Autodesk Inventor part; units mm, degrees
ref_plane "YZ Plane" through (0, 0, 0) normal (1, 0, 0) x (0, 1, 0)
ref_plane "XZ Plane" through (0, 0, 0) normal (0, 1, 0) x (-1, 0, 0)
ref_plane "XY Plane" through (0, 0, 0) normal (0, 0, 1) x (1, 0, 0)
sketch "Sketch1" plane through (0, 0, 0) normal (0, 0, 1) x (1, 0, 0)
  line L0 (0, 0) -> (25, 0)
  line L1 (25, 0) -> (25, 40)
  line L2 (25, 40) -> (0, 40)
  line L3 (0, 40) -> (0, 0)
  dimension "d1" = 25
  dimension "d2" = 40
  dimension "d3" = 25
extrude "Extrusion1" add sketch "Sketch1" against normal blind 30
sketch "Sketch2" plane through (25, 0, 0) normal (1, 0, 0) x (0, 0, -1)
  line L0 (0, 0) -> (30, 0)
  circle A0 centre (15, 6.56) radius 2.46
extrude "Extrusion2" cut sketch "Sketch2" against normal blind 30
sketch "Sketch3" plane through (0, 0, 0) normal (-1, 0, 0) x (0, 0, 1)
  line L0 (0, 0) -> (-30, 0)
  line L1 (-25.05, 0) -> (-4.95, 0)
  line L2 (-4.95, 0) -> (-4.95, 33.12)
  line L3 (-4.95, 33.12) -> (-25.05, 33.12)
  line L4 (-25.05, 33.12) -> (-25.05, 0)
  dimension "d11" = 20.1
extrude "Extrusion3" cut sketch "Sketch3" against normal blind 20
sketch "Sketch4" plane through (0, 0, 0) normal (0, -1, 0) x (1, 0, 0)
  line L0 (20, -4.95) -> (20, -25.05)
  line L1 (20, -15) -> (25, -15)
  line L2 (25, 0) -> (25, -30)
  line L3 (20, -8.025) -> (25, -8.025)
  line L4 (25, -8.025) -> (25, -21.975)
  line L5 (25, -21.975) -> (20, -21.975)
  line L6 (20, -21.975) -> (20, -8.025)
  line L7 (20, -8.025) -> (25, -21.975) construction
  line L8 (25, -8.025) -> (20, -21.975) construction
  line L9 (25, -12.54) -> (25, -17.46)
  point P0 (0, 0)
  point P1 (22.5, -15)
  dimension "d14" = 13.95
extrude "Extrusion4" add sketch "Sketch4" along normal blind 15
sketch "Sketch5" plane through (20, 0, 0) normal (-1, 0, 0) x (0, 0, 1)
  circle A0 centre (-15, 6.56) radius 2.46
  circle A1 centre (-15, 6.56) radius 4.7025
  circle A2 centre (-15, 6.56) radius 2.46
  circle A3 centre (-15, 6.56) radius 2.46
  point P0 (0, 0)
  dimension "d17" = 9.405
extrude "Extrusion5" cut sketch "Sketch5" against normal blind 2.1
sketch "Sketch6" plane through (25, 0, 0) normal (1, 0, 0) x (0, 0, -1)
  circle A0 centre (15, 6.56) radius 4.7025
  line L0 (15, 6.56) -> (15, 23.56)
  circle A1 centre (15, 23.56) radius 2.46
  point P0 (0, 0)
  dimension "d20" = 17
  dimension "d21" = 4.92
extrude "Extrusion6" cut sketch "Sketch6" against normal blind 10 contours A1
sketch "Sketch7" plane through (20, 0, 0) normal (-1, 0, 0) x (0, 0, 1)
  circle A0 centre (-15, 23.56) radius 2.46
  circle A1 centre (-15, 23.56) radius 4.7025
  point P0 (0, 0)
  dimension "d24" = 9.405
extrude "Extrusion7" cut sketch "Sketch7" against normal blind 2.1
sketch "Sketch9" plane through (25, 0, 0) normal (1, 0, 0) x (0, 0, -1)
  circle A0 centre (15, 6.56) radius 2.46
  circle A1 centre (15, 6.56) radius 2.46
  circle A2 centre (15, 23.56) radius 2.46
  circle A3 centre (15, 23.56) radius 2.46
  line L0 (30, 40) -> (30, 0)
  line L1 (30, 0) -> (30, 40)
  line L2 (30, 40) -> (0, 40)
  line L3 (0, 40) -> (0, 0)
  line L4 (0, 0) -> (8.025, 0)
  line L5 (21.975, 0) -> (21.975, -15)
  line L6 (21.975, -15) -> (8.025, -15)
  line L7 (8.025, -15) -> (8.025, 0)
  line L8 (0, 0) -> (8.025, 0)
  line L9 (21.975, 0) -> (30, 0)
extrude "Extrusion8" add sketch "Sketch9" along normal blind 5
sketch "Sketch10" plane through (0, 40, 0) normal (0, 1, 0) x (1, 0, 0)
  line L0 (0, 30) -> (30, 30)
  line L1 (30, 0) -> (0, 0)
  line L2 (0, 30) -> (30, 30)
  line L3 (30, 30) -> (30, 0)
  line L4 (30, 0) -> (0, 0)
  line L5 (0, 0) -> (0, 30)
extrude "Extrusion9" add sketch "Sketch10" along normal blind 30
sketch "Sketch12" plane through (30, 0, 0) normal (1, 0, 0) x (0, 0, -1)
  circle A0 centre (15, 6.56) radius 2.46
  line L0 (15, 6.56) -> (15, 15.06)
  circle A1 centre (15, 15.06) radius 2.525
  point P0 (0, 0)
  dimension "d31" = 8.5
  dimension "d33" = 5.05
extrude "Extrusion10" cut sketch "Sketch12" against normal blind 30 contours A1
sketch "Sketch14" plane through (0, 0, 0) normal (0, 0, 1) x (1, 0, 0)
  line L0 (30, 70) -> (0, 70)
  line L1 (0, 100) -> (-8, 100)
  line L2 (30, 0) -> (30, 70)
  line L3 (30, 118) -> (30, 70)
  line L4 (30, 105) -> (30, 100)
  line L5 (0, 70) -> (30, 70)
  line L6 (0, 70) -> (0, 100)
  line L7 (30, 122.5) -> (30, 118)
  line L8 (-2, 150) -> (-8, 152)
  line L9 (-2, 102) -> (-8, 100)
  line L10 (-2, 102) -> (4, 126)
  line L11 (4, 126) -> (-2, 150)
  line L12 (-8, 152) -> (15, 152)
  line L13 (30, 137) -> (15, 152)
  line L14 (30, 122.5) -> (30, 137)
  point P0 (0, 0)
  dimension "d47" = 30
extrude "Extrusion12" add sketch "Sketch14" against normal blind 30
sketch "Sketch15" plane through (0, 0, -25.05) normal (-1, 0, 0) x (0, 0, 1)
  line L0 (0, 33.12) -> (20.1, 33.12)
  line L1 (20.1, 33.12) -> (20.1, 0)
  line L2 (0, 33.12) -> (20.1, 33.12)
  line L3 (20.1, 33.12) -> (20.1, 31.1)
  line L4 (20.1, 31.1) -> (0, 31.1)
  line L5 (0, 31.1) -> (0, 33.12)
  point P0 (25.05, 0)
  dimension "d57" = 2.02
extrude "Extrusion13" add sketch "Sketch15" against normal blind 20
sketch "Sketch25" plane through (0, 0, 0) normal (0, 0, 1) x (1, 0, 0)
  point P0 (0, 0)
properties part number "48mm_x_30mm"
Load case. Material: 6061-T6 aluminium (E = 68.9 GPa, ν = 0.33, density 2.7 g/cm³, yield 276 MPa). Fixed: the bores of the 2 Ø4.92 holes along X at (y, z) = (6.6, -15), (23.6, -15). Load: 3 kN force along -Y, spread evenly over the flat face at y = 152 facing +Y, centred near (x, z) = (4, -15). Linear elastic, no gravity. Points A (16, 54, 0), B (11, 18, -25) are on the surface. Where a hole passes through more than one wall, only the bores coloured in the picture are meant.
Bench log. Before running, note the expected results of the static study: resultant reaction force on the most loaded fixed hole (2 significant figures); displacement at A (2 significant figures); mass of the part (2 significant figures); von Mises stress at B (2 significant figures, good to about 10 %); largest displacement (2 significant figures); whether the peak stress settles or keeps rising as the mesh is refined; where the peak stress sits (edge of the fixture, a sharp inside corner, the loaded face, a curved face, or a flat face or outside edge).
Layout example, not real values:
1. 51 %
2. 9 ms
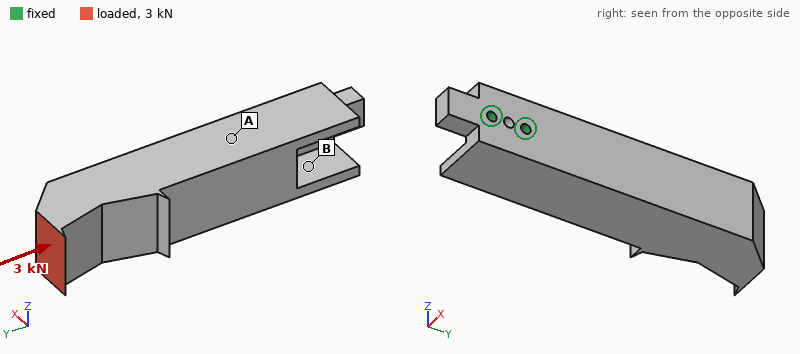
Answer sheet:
1. 3.1 kN
2. 0.049 mm
3. 330 g
4. 22 MPa
5. 0.29 mm
6. keeps rising
7. edge of the fixture
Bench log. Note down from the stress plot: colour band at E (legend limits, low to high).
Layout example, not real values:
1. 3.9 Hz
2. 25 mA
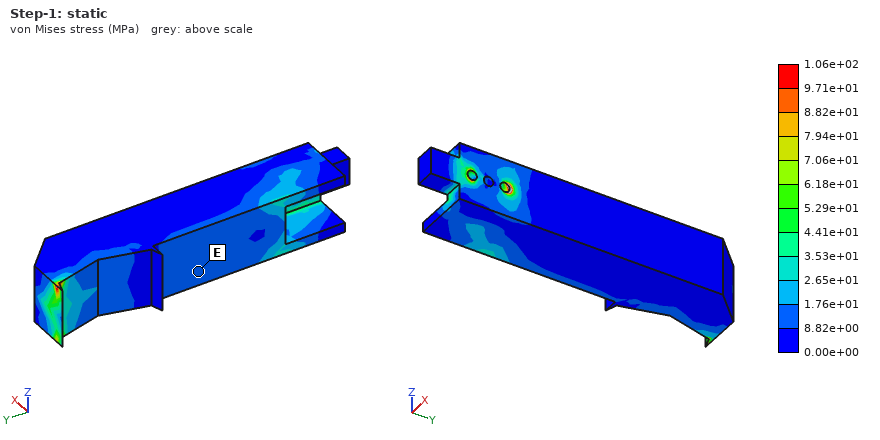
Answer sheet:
1. 8.82e+00 to 1.76e+01 MPa
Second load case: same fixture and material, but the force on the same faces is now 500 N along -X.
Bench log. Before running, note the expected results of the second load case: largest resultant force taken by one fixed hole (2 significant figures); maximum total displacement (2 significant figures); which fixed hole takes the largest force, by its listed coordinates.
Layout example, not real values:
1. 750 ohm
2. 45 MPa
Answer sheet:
1. 3.1 kN
2. 0.26 mm
3. (23.6, -15)
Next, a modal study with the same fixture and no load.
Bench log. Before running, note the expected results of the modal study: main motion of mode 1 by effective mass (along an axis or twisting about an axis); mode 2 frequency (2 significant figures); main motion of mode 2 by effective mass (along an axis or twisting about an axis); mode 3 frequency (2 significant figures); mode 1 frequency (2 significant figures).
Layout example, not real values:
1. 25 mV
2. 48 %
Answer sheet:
1. along X
2. 880 Hz
3. along Z
4. 2900 Hz
5. 760 Hz
